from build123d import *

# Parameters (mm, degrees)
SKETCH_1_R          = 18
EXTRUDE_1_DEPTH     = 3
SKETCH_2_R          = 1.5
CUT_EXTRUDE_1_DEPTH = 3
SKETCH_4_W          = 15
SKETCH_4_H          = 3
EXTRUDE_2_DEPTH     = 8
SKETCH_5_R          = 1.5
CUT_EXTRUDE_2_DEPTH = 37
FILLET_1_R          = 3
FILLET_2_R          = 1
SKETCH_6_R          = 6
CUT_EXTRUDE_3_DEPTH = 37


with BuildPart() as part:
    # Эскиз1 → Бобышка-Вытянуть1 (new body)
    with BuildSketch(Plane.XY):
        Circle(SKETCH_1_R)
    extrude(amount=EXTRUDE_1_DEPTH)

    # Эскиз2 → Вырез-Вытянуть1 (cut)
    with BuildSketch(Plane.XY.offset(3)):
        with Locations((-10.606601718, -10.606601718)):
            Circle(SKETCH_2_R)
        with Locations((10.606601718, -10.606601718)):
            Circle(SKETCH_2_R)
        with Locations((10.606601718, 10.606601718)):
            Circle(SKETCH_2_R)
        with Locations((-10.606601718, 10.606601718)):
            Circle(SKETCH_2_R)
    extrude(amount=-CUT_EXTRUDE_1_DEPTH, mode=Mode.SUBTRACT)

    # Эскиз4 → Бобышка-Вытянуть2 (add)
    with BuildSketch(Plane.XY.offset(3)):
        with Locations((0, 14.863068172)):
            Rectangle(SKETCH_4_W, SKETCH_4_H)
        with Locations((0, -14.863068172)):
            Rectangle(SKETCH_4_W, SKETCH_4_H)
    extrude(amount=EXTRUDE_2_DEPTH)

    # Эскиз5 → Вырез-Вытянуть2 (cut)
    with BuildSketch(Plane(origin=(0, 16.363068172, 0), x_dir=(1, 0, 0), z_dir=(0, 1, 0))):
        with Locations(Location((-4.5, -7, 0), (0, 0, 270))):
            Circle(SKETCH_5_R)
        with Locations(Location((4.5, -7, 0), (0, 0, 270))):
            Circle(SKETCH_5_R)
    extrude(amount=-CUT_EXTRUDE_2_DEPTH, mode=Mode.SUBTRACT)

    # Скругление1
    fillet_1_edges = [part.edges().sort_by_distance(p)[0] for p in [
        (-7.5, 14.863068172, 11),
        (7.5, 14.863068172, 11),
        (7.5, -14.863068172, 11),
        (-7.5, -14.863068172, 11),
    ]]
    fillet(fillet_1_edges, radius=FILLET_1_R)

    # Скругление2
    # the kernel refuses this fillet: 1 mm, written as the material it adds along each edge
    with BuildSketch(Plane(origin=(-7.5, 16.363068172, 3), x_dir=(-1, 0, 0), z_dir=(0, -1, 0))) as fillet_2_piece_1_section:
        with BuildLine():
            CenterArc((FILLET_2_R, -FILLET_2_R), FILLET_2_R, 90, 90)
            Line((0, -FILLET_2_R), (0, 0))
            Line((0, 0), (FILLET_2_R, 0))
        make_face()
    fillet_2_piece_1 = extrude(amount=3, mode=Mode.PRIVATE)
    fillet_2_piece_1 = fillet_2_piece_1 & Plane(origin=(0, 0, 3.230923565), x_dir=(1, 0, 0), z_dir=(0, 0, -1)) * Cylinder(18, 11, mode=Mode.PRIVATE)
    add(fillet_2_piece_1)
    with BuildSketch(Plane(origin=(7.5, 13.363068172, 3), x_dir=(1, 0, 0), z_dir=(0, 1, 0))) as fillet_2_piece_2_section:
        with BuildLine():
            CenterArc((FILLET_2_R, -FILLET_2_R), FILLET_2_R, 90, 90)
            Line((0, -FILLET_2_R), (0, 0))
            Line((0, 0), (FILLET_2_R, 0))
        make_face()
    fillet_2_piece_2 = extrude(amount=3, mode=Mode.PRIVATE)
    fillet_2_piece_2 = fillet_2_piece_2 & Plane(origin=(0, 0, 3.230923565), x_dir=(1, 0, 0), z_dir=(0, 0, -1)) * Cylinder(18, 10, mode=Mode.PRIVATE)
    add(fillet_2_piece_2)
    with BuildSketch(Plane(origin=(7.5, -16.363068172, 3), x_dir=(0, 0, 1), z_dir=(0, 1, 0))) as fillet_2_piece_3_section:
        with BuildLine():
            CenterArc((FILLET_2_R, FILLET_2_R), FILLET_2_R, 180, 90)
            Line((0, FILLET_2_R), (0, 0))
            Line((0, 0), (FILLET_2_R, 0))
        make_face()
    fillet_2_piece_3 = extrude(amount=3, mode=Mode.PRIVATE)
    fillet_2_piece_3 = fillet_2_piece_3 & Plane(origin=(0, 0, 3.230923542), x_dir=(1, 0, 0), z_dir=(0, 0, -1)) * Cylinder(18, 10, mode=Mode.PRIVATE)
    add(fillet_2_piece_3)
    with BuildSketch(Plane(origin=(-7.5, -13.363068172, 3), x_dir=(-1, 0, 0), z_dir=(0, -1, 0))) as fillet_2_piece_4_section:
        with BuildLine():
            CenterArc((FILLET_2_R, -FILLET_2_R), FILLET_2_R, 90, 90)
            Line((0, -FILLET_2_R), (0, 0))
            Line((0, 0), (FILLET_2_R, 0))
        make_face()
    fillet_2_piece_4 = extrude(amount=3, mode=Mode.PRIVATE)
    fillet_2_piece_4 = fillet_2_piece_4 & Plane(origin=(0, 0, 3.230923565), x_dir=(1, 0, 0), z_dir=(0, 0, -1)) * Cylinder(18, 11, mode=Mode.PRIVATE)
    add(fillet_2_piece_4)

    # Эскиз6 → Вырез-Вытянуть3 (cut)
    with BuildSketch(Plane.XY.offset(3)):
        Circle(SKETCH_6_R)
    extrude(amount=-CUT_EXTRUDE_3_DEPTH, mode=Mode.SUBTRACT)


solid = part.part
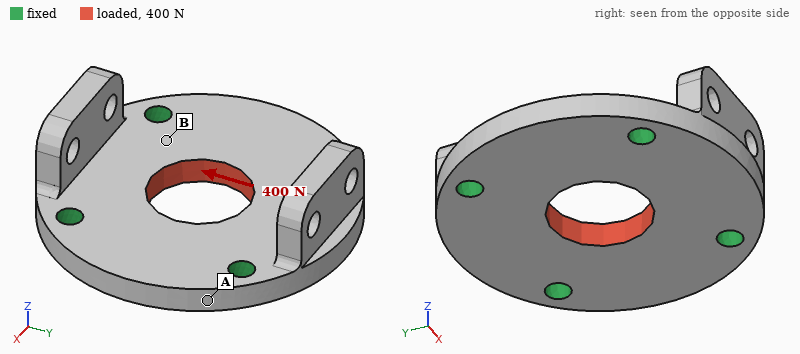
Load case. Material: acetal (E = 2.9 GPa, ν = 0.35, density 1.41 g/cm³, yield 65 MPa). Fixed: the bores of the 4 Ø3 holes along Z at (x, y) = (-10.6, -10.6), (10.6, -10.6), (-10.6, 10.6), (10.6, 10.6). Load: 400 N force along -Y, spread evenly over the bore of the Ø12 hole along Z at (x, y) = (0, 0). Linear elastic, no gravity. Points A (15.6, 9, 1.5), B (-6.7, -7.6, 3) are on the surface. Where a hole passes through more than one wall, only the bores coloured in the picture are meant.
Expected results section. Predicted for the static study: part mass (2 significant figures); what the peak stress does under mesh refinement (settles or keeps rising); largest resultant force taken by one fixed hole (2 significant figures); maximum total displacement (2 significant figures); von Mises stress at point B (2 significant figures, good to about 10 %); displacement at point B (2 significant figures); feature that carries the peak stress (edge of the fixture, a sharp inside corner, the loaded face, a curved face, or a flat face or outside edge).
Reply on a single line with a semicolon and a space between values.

4.6 g; keeps rising; 100 N; 21 µm; 4.1 MPa; 9.1 µm; edge of the fixture
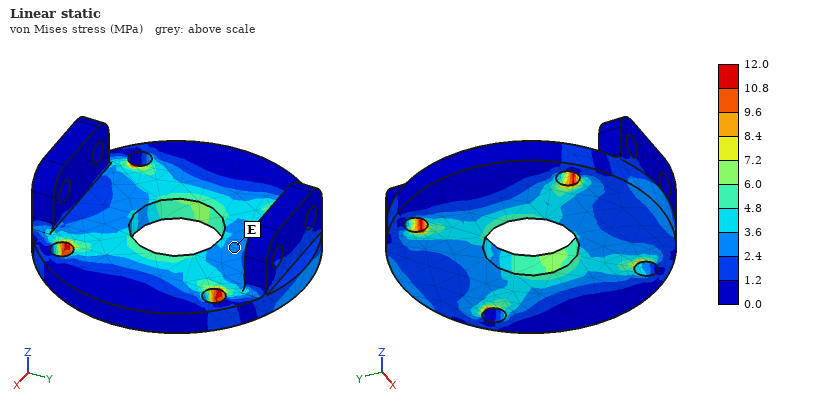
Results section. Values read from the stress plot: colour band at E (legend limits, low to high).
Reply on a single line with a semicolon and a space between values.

2.4 to 3.6 MPa
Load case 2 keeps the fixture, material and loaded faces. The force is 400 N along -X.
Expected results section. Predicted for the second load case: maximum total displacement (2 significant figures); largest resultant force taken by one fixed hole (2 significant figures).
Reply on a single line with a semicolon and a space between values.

21 µm; 100 N
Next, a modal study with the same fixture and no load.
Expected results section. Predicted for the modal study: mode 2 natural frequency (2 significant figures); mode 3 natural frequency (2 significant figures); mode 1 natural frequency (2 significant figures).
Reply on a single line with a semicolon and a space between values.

4800 Hz; 8000 Hz; 4600 Hz
